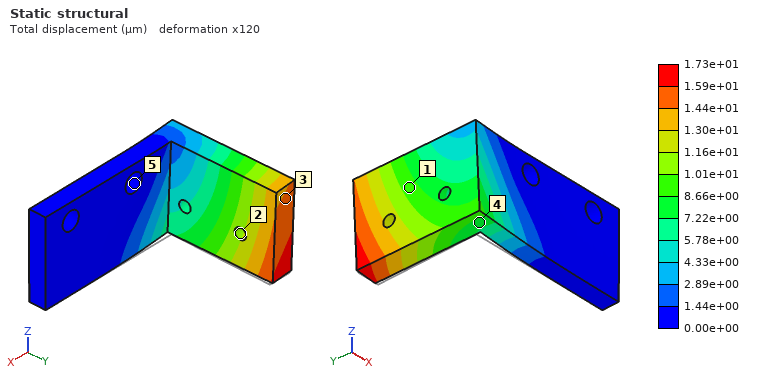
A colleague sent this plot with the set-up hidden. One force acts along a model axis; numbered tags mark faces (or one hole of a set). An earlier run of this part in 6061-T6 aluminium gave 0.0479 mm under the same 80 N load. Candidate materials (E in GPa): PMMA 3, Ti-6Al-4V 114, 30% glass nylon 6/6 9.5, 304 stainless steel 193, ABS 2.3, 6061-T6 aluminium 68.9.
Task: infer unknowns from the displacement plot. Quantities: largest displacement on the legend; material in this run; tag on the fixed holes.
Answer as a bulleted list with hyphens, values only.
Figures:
- 1.73e+01 µm
- 304 stainless steel
- 5
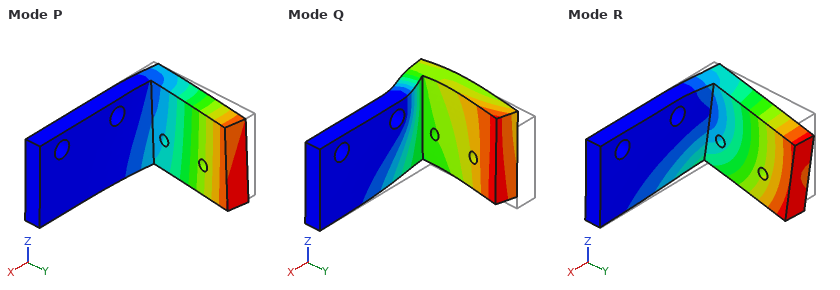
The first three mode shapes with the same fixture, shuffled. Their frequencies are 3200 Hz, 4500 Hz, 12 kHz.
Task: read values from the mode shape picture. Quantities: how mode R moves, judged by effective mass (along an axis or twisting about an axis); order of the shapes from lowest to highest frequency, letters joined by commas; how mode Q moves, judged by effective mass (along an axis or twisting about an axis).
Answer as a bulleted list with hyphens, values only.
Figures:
- along Z
- P, R, Q
- along Y
